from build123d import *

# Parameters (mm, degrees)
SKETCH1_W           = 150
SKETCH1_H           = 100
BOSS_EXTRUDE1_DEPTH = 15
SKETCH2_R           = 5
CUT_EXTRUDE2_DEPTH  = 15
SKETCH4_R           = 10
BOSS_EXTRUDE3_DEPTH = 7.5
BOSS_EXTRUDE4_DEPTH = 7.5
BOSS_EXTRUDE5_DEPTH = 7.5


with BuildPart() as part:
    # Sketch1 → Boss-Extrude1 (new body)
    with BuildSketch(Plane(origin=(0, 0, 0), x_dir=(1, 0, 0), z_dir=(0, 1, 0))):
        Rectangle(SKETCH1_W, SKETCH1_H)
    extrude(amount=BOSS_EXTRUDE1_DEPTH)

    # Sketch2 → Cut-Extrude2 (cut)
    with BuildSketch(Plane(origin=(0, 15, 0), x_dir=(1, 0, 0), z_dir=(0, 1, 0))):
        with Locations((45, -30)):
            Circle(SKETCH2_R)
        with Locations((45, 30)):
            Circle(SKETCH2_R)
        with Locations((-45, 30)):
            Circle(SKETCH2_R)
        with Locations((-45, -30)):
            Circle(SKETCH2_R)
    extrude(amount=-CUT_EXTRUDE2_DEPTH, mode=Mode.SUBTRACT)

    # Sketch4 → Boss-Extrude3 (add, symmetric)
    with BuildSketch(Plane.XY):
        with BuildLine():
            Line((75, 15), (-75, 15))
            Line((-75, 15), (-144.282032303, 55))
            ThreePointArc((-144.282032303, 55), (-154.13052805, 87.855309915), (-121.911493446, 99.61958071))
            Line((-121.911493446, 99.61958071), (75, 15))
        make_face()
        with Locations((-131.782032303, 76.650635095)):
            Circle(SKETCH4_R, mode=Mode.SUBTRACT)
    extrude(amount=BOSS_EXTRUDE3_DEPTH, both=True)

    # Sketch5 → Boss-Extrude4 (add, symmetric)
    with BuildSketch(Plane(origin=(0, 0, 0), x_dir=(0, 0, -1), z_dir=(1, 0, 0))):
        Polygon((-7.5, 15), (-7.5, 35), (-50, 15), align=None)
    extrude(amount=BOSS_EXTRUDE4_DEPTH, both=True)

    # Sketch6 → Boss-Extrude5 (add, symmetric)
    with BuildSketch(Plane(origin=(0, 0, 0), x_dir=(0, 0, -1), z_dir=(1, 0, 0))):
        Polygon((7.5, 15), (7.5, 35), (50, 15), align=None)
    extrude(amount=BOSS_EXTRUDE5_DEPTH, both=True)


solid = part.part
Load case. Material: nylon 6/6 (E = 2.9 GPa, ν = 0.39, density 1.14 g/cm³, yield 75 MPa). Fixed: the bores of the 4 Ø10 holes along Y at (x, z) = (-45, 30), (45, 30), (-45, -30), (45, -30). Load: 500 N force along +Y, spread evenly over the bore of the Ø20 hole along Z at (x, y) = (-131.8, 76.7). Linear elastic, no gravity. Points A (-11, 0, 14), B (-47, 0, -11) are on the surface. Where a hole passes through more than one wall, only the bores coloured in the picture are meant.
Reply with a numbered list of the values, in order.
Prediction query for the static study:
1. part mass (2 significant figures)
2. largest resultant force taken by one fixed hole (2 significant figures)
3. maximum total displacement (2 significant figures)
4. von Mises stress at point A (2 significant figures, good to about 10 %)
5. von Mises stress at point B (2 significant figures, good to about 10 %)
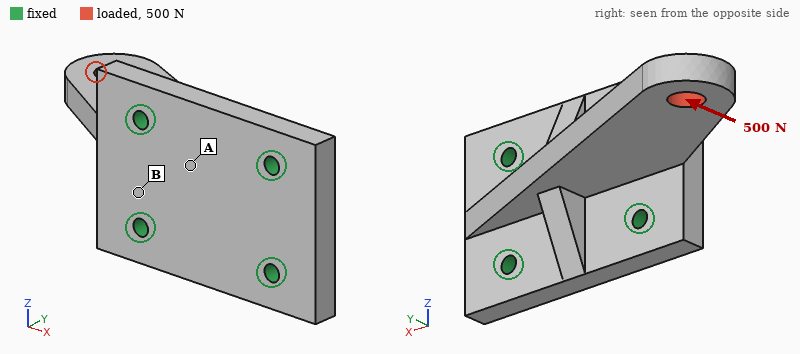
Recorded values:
1. 420 g
2. 510 N
3. 0.55 mm
4. 0.72 MPa
5. 2.0 MPa
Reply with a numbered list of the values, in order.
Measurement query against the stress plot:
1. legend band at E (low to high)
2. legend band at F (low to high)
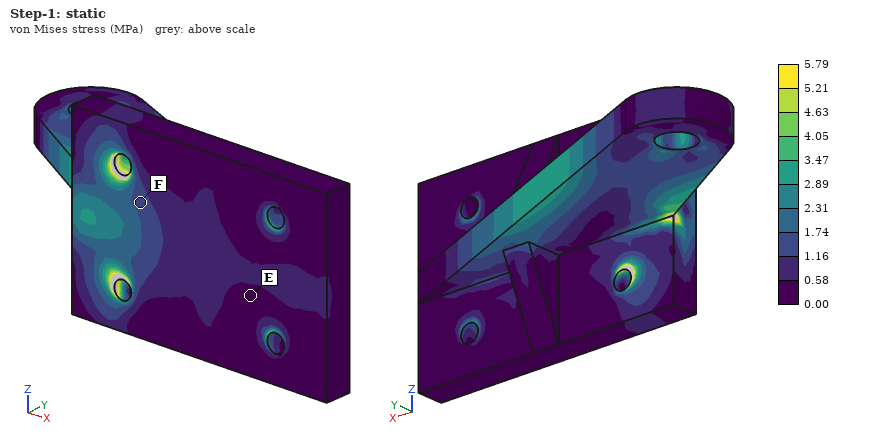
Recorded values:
1. 0.00 to 0.58 MPa
2. 1.16 to 1.74 MPa
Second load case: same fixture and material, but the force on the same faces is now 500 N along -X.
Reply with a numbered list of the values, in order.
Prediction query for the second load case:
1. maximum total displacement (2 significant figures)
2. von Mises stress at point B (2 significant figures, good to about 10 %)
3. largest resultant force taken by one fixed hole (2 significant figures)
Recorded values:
1. 0.32 mm
2. 0.86 MPa
3. 250 N
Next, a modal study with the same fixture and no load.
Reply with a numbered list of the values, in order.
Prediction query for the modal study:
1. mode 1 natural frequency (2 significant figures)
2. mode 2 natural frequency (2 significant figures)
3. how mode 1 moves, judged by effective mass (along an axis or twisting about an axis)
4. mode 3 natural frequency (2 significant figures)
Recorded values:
1. 290 Hz
2. 740 Hz
3. along Z
4. 990 Hz
